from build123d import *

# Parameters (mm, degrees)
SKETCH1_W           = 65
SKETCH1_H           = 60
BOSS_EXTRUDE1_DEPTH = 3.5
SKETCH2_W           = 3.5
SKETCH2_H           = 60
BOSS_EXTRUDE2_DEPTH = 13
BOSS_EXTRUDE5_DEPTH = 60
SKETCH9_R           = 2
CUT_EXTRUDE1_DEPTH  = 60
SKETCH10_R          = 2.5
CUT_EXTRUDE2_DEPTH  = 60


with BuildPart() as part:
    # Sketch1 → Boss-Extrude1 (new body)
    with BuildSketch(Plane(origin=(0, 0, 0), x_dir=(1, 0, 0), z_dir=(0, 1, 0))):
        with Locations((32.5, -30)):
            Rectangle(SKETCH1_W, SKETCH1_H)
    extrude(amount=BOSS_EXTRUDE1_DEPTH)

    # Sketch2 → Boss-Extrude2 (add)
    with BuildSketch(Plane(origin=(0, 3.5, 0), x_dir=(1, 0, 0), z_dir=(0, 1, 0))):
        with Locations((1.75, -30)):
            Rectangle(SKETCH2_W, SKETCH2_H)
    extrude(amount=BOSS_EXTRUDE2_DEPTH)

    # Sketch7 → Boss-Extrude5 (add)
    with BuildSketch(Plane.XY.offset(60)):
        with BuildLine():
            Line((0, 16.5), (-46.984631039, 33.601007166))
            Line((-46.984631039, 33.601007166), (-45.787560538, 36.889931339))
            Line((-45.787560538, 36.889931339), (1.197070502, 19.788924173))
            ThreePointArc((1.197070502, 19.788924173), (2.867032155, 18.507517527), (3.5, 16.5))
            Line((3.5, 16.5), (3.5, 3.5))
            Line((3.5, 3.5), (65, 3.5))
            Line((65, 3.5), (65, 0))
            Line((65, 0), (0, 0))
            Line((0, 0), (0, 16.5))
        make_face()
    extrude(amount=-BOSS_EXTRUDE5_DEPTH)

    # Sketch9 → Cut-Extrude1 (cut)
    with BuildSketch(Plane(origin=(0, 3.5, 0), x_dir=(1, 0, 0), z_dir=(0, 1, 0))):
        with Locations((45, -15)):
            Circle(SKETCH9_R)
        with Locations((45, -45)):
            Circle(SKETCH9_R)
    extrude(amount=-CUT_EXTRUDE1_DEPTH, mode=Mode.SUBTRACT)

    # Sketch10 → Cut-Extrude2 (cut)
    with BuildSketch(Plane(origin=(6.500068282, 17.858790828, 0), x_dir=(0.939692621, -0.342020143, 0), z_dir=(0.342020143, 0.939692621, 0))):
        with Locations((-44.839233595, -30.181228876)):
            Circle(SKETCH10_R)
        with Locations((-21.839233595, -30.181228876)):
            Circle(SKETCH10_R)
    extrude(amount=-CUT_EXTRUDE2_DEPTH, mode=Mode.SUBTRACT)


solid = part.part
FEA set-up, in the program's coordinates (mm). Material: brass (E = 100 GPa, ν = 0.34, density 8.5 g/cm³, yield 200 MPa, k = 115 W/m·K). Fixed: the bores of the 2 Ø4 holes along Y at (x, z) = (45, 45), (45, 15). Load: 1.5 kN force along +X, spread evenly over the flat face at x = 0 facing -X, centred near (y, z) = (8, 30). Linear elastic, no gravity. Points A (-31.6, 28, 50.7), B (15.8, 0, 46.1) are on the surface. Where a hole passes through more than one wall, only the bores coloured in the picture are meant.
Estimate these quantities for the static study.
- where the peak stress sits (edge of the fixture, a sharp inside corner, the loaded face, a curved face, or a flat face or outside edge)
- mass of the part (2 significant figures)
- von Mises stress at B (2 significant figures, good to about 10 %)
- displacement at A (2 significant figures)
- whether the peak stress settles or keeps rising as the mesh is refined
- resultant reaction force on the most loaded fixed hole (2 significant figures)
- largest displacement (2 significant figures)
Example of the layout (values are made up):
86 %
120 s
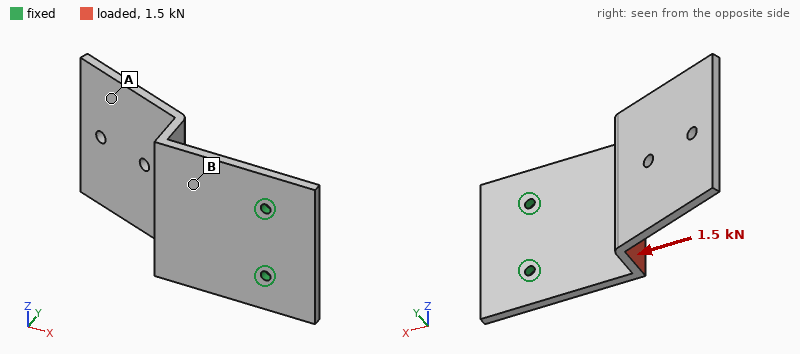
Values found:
edge of the fixture
230 g
64 MPa
1.2 mm
keeps rising
760 N
1.6 mm
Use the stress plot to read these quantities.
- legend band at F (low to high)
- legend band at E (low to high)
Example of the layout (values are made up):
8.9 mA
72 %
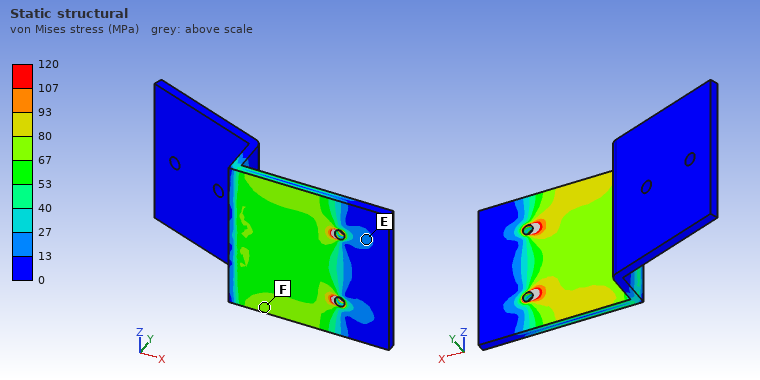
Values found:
67 to 80 MPa
13 to 27 MPa
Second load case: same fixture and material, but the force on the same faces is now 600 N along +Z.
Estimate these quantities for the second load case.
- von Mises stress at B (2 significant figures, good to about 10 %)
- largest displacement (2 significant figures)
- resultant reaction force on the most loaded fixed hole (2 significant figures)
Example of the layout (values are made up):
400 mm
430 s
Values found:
13 MPa
0.14 mm
900 N
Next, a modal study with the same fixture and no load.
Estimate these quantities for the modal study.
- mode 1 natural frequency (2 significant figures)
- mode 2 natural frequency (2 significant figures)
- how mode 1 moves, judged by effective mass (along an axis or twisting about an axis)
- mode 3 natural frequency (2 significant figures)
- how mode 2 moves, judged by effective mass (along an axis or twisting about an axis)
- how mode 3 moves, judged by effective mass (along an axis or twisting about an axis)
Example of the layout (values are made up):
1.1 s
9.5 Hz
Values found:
190 Hz
570 Hz
along Y
960 Hz
along Z
along Y
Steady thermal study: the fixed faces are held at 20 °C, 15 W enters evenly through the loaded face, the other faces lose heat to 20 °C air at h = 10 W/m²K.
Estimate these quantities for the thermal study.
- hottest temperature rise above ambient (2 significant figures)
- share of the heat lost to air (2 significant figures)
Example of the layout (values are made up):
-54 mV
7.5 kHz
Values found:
27 K
18 %
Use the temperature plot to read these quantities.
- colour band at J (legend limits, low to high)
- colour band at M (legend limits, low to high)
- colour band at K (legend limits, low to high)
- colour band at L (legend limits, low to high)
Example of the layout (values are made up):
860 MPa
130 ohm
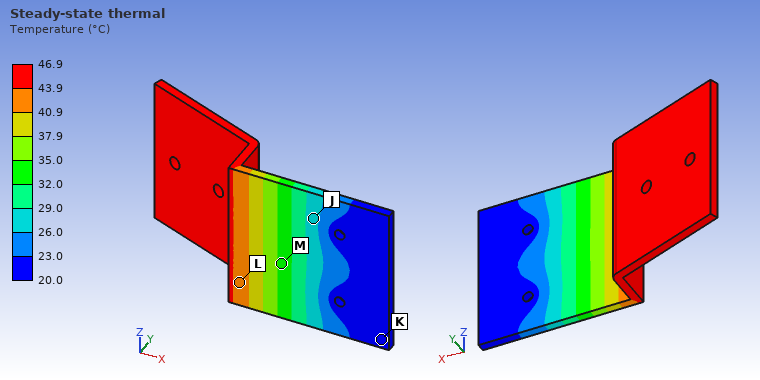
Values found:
26.0 to 29.0 °C
32.0 to 35.0 °C
20.0 to 23.0 °C
40.9 to 43.9 °C
